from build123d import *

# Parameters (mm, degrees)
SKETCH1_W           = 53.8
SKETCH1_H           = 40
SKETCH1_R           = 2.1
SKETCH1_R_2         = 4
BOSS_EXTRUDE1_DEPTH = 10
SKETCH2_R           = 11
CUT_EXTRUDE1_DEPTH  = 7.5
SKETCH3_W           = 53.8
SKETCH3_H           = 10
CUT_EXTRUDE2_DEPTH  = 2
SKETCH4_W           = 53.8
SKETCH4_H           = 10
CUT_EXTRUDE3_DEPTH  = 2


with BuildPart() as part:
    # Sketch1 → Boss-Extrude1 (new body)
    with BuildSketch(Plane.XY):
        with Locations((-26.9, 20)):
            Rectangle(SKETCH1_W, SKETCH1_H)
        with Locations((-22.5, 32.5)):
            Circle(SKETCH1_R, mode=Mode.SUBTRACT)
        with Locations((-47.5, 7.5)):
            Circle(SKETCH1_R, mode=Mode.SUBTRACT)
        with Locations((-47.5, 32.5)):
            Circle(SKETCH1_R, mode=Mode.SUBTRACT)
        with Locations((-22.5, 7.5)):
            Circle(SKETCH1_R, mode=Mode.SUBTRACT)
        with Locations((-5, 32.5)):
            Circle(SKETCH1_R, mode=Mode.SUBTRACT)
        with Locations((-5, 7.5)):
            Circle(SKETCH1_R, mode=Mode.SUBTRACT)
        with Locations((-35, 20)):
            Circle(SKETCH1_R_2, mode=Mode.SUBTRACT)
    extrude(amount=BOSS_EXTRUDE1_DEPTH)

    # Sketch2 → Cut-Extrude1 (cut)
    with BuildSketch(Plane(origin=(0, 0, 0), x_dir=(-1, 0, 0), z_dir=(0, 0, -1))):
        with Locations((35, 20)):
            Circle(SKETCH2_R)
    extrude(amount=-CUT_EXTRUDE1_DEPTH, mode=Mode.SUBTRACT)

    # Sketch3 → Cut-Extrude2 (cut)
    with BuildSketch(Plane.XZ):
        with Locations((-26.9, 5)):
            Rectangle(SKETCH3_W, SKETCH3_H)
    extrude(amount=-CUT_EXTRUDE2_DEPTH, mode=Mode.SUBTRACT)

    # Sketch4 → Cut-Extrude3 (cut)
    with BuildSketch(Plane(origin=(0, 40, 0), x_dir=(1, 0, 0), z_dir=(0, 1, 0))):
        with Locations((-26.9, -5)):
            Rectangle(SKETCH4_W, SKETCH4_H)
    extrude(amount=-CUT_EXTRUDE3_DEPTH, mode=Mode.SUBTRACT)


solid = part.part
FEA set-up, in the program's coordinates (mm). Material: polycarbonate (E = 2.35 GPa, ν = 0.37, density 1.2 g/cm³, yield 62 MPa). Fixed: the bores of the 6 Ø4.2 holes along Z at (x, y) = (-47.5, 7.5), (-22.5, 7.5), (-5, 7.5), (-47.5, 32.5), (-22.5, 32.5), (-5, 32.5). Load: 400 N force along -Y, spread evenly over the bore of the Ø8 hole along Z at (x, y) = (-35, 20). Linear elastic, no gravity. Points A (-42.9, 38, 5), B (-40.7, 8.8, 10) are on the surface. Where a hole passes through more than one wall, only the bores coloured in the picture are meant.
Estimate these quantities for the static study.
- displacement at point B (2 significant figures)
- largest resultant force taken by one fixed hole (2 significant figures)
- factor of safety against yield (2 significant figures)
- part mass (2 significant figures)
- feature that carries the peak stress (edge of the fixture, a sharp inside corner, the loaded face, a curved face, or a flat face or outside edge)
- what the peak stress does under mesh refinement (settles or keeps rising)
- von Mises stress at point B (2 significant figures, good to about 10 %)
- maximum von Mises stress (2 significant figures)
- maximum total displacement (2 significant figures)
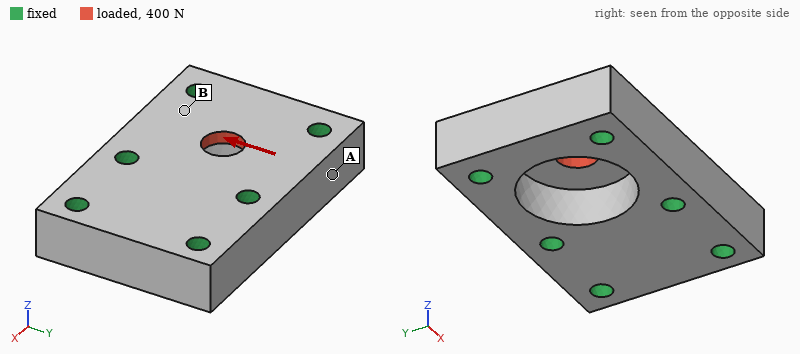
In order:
12 µm
110 N
5.4
19 g
the loaded face
settles
3.4 MPa
11 MPa
31 µm
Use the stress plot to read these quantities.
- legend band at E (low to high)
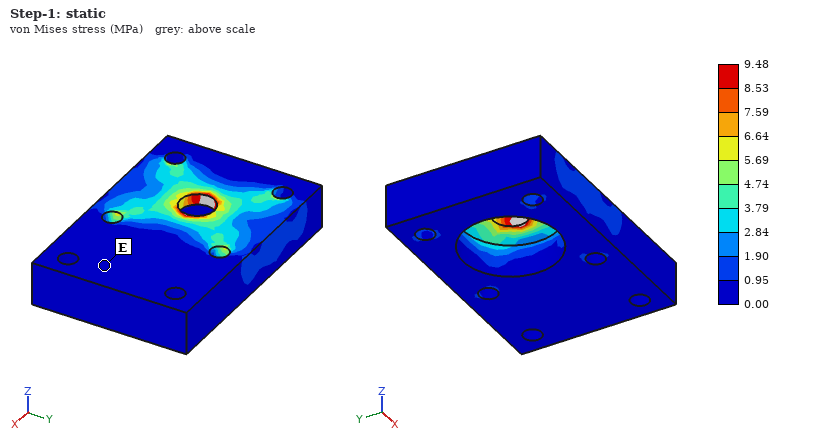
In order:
0.00 to 0.95 MPa
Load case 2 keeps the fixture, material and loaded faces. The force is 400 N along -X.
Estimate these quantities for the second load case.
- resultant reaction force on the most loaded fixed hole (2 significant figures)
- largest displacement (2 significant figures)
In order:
100 N
30 µm
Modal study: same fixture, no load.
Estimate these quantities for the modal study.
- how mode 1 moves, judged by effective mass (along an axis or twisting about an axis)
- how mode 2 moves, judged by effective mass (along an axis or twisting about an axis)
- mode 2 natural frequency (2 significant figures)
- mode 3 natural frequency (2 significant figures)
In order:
along Z
along Z
13 kHz
14 kHz
